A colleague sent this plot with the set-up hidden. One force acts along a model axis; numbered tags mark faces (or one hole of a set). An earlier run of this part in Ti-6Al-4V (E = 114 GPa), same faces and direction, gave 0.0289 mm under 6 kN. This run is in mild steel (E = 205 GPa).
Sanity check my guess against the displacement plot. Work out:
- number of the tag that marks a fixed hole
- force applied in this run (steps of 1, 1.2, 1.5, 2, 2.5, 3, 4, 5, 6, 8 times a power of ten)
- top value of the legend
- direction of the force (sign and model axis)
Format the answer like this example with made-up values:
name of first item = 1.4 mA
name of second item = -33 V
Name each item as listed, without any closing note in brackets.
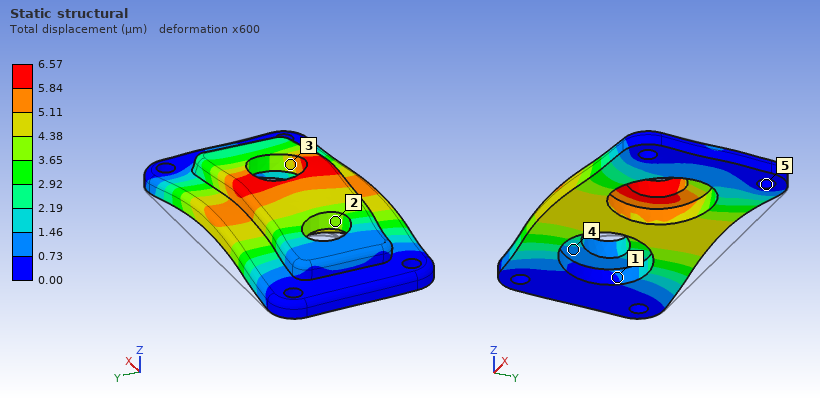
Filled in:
number of the tag that marks a fixed hole = 5
force applied in this run = 2.5 kN
top value of the legend = 6.57 µm
direction of the force = -Y
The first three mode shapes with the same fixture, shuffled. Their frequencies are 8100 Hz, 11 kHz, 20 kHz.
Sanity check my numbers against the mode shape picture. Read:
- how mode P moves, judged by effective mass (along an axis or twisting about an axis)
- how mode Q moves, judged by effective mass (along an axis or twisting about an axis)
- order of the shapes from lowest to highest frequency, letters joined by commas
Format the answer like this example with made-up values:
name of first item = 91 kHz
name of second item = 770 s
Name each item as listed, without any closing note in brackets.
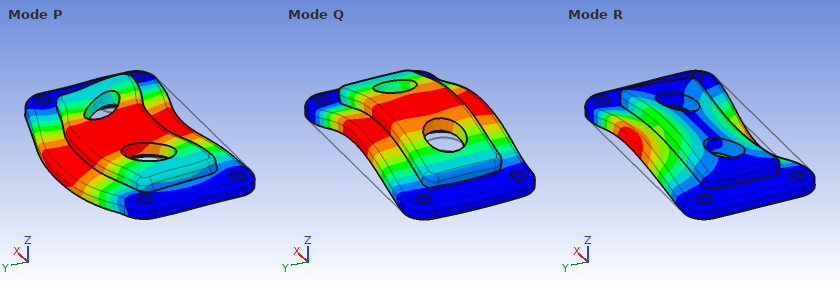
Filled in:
how mode P moves, judged by effective mass = along Y
how mode Q moves, judged by effective mass = along Z
order of the shapes from lowest to highest frequency, letters joined by commas = Q, R, P
